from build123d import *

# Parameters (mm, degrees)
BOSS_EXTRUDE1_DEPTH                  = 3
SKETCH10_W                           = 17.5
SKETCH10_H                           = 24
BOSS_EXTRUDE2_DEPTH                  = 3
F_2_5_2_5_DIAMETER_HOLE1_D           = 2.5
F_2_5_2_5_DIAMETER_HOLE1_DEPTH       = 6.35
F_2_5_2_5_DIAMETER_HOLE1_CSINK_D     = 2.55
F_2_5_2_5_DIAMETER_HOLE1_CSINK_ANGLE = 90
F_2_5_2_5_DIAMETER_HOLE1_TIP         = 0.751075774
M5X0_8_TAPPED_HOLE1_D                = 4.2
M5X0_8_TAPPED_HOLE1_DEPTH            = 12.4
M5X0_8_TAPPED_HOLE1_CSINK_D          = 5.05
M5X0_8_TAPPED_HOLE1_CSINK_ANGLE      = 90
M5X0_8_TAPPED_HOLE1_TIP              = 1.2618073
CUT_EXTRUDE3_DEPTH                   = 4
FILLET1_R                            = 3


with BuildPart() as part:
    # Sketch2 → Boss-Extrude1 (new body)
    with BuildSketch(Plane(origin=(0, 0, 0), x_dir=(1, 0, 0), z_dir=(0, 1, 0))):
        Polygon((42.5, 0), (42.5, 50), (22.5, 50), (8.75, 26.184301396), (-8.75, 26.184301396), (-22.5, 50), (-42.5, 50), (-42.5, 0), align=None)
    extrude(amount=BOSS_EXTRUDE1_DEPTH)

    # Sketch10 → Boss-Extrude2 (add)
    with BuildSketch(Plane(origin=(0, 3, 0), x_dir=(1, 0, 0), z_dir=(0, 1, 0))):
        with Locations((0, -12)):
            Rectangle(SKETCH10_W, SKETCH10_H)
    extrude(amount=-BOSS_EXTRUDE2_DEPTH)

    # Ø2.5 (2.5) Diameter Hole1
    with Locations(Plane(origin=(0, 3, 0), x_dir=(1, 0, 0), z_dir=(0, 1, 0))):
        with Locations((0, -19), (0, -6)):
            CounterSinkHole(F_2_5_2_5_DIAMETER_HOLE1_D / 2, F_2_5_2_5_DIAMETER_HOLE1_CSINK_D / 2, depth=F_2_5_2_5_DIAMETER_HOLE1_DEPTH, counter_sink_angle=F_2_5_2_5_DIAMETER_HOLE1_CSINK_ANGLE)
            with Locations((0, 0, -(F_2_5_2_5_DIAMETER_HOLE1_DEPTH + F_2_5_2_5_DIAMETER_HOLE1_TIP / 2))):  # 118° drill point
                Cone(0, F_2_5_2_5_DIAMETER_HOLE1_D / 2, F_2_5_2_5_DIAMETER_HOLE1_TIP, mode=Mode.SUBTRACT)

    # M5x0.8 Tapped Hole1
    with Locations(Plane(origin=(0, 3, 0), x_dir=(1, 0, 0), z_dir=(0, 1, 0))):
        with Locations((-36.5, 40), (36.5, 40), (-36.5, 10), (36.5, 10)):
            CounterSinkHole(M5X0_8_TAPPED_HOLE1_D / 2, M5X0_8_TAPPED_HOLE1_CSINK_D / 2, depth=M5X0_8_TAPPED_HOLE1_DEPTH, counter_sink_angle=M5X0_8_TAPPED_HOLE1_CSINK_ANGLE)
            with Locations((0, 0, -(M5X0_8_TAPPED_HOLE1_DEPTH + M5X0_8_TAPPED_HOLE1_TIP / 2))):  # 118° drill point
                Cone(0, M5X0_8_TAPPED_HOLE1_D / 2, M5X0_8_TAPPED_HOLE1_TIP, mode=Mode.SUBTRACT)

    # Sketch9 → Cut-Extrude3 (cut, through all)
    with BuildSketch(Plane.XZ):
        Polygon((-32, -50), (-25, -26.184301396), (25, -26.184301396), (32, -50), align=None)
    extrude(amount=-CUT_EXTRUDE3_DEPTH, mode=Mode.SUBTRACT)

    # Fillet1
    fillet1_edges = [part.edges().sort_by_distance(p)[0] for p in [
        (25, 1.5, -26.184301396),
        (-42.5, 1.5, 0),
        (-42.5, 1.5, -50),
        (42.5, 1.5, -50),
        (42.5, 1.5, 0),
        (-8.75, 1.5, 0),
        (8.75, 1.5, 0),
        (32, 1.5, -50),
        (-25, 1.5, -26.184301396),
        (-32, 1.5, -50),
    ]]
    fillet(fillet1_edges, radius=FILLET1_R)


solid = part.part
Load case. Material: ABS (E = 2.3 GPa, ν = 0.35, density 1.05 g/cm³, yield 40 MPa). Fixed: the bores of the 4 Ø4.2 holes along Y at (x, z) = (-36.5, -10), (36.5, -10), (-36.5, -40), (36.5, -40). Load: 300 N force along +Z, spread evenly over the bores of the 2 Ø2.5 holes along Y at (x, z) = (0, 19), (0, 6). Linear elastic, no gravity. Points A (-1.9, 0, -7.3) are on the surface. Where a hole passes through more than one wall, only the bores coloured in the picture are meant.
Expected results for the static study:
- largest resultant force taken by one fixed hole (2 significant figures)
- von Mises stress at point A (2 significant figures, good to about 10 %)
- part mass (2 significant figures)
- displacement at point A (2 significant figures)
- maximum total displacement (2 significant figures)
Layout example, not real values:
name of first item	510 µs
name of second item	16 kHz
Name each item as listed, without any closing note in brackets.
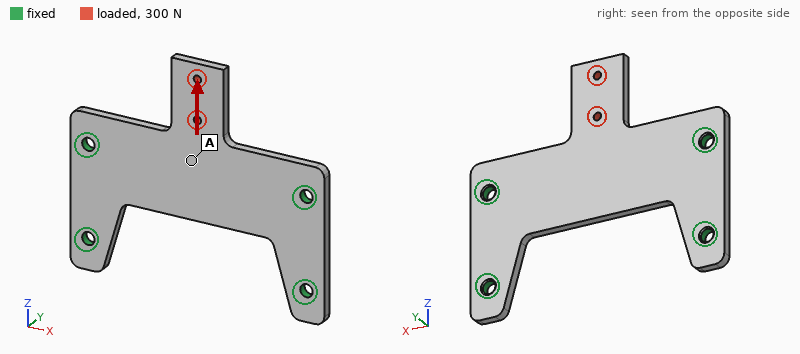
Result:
largest resultant force taken by one fixed hole	100 N
von Mises stress at point A	2.5 MPa
part mass	10 g
displacement at point A	0.12 mm
maximum total displacement	0.17 mm
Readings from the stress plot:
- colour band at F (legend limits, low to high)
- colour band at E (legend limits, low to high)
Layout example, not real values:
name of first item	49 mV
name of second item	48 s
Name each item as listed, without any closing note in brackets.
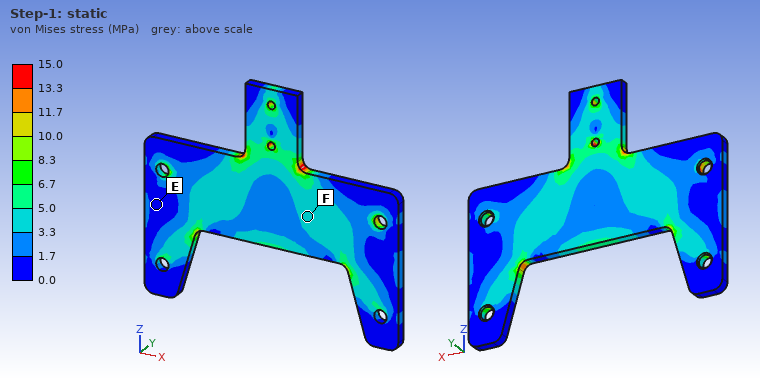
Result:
colour band at F	3.3 to 5.0 MPa
colour band at E	0.0 to 1.7 MPa
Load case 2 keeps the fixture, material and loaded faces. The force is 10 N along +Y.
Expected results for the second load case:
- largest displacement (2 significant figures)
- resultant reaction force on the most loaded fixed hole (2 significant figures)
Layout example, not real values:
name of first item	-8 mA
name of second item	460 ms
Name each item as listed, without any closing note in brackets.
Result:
largest displacement	1.2 mm
resultant reaction force on the most loaded fixed hole	7.8 N
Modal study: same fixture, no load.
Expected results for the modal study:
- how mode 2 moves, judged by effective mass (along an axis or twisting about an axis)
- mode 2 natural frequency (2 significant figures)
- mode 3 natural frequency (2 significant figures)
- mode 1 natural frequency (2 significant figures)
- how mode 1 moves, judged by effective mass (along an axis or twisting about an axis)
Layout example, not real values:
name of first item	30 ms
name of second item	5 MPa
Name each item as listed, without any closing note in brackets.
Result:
how mode 2 moves, judged by effective mass	along Y
mode 2 natural frequency	950 Hz
mode 3 natural frequency	2000 Hz
mode 1 natural frequency	470 Hz
how mode 1 moves, judged by effective mass	along Y
